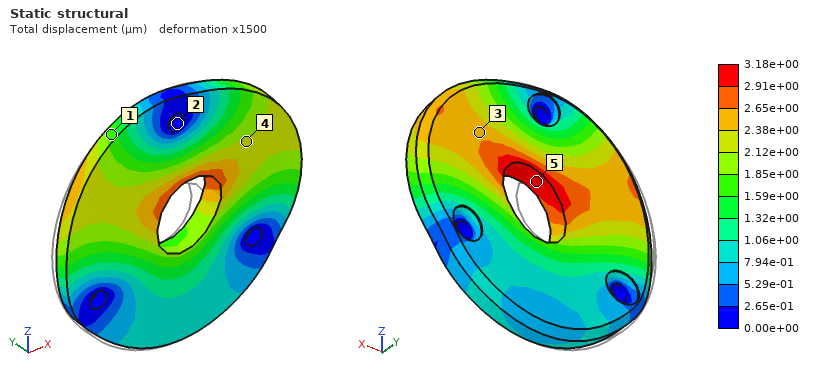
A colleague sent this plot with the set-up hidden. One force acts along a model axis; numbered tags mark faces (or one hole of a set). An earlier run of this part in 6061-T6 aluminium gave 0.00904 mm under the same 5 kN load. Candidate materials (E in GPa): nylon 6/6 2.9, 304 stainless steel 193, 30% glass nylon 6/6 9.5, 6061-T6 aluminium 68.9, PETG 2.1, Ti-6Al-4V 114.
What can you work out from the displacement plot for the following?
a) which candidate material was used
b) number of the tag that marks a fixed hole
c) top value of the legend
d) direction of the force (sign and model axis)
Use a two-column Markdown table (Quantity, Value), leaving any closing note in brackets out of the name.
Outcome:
| Quantity | Value |
|---|---|
| which candidate material was used | 304 stainless steel |
| number of the tag that marks a fixed hole | 2 |
| top value of the legend | 3.18e+00 µm |
| direction of the force | +X |
